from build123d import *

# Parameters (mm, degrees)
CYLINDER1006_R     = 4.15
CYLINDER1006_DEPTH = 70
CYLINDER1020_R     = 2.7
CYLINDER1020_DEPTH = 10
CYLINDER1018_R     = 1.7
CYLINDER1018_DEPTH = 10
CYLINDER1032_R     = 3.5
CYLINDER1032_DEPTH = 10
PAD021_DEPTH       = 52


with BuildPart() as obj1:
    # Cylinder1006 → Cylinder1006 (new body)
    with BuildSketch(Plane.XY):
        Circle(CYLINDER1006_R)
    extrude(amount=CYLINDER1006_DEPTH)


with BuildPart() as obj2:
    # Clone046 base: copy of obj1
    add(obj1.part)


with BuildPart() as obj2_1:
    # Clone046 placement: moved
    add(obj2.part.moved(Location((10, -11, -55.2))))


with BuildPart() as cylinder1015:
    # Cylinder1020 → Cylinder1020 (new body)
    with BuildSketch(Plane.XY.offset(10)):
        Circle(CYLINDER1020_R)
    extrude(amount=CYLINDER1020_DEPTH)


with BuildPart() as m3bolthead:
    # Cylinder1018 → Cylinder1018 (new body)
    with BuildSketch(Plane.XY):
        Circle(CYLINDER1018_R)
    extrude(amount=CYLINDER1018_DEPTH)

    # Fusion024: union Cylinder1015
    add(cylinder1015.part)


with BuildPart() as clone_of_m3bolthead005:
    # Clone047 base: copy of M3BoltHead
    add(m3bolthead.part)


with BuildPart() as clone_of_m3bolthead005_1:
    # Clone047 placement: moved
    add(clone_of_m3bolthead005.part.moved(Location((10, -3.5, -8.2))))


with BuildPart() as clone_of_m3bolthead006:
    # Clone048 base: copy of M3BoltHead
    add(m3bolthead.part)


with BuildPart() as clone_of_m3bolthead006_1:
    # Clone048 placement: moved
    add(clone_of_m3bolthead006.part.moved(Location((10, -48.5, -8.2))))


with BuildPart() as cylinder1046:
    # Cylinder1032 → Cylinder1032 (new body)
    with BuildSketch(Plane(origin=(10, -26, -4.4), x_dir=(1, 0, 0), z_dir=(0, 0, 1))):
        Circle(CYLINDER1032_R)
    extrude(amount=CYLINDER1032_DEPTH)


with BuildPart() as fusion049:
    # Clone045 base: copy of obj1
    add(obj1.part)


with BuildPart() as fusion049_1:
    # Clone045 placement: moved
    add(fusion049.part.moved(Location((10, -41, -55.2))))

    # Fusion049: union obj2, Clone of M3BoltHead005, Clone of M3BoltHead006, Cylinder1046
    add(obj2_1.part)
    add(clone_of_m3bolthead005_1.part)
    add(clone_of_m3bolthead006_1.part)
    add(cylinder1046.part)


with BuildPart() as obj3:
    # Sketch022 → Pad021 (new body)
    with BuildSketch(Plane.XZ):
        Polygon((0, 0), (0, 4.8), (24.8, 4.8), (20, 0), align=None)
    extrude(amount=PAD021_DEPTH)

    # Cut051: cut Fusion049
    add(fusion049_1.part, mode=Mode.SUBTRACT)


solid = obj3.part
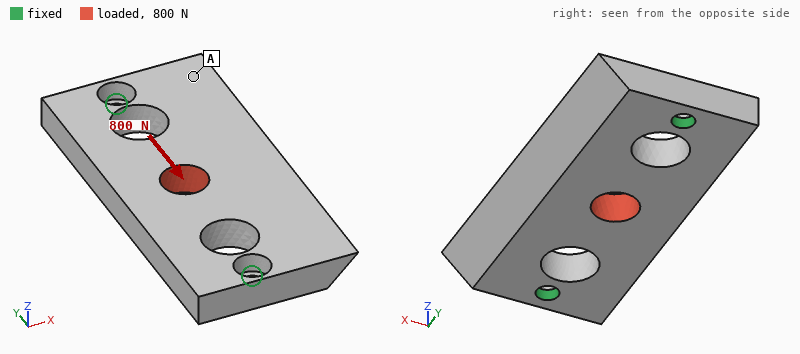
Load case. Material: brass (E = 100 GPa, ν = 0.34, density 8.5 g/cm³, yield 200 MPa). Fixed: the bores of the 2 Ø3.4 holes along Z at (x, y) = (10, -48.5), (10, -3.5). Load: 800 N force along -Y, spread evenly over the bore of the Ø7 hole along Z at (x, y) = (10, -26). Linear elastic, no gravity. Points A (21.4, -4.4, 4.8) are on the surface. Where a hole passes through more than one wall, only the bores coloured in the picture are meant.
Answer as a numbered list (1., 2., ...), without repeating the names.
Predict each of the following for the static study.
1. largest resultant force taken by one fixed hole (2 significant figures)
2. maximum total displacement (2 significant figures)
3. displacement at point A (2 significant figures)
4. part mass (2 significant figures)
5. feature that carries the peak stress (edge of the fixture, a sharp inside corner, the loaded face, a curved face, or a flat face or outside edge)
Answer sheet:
1. 400 N
2. 3.9 µm
3. 2.9 µm
4. 40 g
5. edge of the fixture
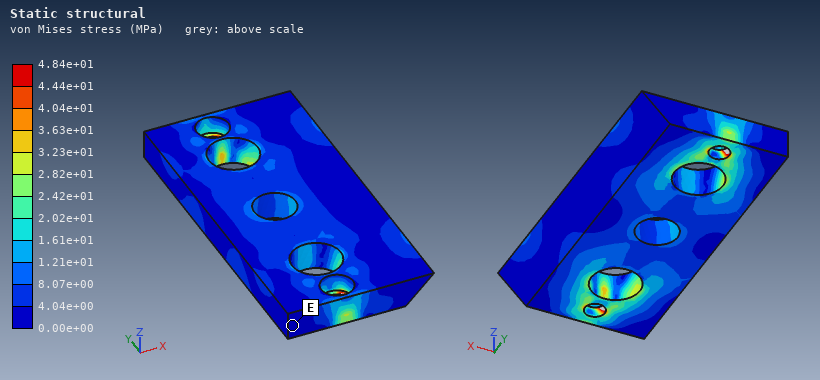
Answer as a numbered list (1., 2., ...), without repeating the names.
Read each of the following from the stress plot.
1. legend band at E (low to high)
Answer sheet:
1. 0.00e+00 to 4.04e+00 MPa
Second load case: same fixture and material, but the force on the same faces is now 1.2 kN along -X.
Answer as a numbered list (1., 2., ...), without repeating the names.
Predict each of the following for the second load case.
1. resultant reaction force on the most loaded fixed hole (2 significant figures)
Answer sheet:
1. 600 N
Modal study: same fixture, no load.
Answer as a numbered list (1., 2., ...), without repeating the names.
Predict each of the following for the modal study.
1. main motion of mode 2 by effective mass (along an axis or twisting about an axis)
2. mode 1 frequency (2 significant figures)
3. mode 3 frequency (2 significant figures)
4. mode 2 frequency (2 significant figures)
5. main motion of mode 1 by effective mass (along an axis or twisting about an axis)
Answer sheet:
1. along Z
2. 4000 Hz
3. 9200 Hz
4. 4900 Hz
5. along Z
